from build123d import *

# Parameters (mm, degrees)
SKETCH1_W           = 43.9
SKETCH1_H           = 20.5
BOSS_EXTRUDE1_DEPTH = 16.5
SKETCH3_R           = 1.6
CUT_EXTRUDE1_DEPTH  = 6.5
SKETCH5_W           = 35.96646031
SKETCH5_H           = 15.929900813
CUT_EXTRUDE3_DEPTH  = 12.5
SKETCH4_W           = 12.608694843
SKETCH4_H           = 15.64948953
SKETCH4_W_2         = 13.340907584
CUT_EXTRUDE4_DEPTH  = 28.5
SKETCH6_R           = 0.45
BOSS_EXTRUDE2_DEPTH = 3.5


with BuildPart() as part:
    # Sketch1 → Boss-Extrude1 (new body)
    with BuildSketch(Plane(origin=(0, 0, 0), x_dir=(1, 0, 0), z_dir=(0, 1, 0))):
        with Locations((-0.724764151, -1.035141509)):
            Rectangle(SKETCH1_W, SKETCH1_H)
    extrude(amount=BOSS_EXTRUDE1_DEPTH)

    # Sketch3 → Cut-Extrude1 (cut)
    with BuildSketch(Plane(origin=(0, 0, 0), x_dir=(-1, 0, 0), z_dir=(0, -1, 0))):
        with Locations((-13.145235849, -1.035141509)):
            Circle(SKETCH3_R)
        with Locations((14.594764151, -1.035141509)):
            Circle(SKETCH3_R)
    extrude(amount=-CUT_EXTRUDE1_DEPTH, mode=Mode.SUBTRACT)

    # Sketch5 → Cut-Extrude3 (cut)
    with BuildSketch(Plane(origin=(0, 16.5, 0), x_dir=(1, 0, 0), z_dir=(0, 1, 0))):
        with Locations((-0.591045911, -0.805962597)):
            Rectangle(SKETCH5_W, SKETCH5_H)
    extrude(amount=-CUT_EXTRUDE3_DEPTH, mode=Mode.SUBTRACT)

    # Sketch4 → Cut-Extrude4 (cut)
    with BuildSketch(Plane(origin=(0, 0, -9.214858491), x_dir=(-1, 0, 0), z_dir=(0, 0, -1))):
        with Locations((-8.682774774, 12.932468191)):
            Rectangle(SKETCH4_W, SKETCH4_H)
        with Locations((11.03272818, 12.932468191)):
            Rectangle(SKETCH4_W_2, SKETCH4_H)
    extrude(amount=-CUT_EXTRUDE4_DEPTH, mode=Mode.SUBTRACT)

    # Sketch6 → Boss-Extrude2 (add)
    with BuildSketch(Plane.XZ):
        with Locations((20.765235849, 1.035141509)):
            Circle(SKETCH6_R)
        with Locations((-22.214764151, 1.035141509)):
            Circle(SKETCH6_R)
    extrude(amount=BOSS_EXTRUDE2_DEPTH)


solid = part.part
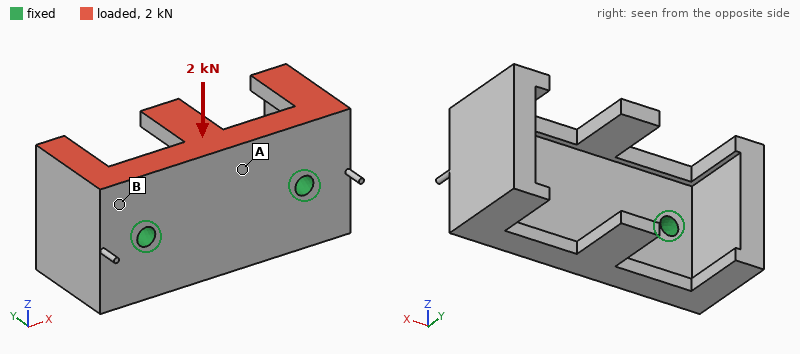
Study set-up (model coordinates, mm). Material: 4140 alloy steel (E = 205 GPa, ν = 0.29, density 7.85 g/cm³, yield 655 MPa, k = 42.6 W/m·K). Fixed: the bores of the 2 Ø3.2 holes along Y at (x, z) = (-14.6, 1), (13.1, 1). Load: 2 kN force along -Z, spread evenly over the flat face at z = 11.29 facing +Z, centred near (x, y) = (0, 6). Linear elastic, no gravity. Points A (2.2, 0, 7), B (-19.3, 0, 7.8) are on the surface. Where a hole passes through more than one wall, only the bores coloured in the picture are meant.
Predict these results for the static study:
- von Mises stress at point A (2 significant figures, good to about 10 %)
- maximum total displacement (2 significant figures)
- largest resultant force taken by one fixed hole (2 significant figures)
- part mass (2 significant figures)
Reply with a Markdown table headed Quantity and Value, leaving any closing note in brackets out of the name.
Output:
| Quantity | Value |
|---|---|
| von Mises stress at point A | 47 MPa |
| maximum total displacement | 91 µm |
| largest resultant force taken by one fixed hole | 1.0 kN |
| part mass | 49 g |
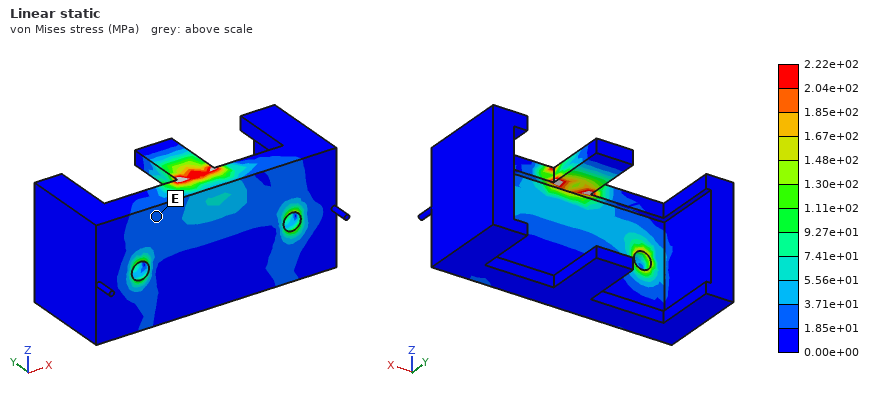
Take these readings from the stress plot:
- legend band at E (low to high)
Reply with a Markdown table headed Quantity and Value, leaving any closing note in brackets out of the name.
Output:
| Quantity | Value |
|---|---|
| legend band at E | 1.85e+01 to 3.71e+01 MPa |
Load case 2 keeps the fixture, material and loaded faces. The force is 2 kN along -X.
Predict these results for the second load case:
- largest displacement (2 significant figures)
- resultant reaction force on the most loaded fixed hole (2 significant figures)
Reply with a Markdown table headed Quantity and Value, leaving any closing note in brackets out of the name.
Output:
| Quantity | Value |
|---|---|
| largest displacement | 20 µm |
| resultant reaction force on the most loaded fixed hole | 1.2 kN |
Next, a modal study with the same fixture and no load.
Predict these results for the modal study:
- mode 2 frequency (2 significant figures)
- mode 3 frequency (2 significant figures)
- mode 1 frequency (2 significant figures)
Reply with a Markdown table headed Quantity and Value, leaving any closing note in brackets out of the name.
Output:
| Quantity | Value |
|---|---|
| mode 2 frequency | 9500 Hz |
| mode 3 frequency | 10 kHz |
| mode 1 frequency | 8800 Hz |
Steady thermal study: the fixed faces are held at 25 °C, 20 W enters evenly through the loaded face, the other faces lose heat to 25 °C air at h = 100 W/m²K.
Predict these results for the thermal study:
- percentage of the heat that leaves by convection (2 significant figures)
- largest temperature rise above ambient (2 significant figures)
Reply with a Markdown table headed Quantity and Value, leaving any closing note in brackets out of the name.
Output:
| Quantity | Value |
|---|---|
| percentage of the heat that leaves by convection | 25 % |
| largest temperature rise above ambient | 56 K |
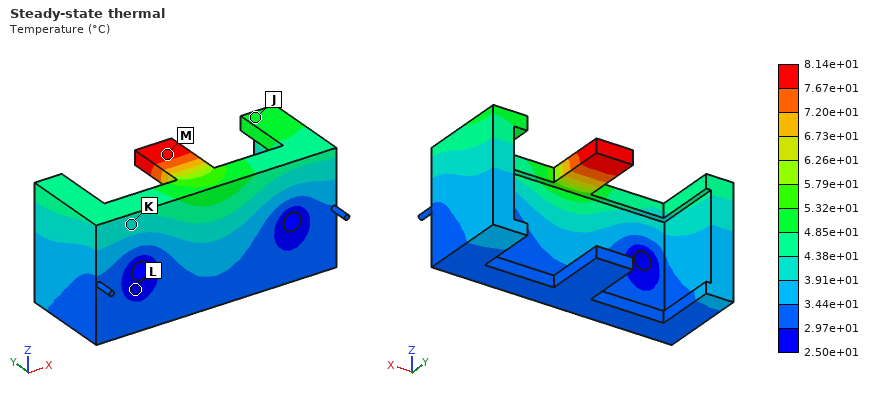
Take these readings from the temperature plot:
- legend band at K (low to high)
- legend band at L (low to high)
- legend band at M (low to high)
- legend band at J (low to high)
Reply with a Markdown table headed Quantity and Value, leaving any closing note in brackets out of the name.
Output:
| Quantity | Value |
|---|---|
| legend band at K | 3.91e+01 to 4.38e+01 °C |
| legend band at L | 2.50e+01 to 2.97e+01 °C |
| legend band at M | 7.67e+01 to 8.14e+01 °C |
| legend band at J | 4.85e+01 to 5.32e+01 °C |
